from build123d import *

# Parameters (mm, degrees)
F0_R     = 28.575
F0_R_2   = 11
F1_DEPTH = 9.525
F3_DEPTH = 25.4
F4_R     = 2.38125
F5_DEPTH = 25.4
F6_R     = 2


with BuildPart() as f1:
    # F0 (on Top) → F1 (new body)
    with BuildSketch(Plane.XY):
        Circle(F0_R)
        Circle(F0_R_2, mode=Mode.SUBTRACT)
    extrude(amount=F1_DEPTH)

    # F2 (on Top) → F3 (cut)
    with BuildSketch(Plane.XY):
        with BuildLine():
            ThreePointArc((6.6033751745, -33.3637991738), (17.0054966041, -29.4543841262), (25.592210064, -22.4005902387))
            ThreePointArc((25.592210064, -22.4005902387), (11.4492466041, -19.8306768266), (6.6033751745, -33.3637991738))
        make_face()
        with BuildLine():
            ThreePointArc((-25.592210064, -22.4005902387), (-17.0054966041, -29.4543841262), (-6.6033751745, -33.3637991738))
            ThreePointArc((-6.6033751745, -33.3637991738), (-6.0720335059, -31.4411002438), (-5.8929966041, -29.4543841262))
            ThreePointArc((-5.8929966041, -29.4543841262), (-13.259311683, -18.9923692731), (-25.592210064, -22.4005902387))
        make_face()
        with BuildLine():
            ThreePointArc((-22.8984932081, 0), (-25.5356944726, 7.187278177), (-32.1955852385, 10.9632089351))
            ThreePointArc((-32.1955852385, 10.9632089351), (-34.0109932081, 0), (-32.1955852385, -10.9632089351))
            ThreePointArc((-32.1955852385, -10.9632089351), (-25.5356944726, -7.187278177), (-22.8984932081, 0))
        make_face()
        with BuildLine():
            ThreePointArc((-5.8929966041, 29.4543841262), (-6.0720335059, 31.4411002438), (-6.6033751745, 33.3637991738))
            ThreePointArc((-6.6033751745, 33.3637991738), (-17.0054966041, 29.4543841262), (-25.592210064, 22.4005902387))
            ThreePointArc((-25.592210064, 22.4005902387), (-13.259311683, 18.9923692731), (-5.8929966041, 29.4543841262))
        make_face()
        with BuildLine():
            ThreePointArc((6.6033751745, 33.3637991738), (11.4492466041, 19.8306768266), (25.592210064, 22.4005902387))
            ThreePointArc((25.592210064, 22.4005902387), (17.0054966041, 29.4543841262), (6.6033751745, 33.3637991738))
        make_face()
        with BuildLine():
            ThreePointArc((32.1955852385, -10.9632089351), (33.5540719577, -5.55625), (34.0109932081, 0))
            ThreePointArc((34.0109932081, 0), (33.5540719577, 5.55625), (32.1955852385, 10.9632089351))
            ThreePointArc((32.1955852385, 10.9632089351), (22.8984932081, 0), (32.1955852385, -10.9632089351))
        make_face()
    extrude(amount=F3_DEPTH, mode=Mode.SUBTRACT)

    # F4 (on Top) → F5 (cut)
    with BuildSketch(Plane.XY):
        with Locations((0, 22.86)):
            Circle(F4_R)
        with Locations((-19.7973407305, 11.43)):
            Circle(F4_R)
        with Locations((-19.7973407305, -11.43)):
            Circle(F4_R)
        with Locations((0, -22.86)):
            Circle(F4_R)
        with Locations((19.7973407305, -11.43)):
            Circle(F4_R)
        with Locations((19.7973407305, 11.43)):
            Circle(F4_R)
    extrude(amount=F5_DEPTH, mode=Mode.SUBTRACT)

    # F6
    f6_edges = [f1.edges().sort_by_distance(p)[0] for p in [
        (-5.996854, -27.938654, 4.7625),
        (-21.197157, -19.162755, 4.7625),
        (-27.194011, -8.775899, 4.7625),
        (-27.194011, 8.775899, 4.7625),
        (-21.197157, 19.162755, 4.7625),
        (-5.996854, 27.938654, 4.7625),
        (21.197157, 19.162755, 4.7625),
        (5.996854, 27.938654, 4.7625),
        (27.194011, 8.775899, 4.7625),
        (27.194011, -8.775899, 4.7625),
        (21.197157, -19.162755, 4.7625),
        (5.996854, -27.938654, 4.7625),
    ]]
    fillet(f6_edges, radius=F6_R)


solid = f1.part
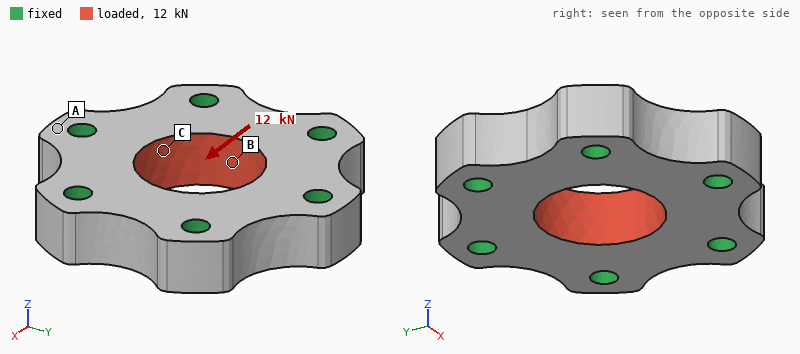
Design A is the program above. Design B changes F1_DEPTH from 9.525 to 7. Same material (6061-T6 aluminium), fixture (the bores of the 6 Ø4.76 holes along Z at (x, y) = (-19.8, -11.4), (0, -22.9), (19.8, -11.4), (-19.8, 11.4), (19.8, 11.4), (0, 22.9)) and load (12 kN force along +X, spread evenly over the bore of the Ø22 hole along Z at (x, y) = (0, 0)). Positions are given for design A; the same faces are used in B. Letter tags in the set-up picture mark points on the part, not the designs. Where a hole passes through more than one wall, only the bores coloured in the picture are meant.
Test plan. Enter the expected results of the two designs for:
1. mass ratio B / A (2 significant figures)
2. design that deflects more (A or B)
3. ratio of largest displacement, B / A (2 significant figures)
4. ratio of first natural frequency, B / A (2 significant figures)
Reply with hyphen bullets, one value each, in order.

- 0.73
- B
- 1.4
- 0.88
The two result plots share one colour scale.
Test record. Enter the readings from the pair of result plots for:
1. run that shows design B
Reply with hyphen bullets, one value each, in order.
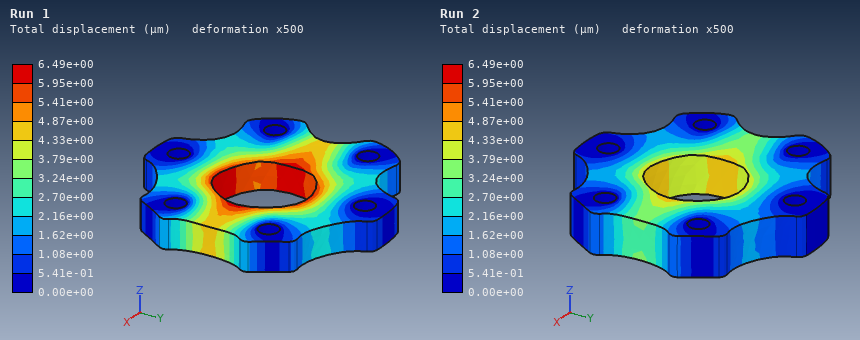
- Run 1
